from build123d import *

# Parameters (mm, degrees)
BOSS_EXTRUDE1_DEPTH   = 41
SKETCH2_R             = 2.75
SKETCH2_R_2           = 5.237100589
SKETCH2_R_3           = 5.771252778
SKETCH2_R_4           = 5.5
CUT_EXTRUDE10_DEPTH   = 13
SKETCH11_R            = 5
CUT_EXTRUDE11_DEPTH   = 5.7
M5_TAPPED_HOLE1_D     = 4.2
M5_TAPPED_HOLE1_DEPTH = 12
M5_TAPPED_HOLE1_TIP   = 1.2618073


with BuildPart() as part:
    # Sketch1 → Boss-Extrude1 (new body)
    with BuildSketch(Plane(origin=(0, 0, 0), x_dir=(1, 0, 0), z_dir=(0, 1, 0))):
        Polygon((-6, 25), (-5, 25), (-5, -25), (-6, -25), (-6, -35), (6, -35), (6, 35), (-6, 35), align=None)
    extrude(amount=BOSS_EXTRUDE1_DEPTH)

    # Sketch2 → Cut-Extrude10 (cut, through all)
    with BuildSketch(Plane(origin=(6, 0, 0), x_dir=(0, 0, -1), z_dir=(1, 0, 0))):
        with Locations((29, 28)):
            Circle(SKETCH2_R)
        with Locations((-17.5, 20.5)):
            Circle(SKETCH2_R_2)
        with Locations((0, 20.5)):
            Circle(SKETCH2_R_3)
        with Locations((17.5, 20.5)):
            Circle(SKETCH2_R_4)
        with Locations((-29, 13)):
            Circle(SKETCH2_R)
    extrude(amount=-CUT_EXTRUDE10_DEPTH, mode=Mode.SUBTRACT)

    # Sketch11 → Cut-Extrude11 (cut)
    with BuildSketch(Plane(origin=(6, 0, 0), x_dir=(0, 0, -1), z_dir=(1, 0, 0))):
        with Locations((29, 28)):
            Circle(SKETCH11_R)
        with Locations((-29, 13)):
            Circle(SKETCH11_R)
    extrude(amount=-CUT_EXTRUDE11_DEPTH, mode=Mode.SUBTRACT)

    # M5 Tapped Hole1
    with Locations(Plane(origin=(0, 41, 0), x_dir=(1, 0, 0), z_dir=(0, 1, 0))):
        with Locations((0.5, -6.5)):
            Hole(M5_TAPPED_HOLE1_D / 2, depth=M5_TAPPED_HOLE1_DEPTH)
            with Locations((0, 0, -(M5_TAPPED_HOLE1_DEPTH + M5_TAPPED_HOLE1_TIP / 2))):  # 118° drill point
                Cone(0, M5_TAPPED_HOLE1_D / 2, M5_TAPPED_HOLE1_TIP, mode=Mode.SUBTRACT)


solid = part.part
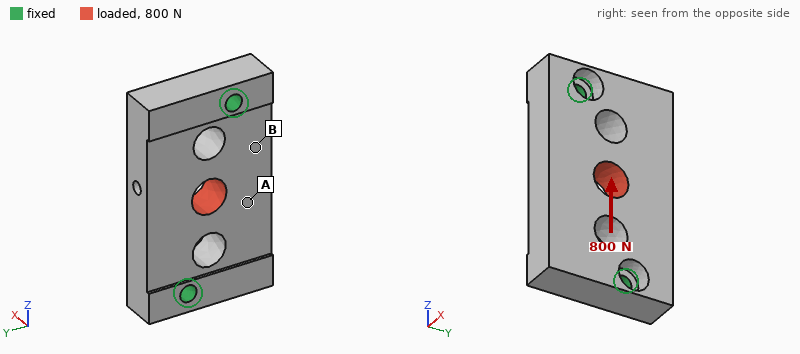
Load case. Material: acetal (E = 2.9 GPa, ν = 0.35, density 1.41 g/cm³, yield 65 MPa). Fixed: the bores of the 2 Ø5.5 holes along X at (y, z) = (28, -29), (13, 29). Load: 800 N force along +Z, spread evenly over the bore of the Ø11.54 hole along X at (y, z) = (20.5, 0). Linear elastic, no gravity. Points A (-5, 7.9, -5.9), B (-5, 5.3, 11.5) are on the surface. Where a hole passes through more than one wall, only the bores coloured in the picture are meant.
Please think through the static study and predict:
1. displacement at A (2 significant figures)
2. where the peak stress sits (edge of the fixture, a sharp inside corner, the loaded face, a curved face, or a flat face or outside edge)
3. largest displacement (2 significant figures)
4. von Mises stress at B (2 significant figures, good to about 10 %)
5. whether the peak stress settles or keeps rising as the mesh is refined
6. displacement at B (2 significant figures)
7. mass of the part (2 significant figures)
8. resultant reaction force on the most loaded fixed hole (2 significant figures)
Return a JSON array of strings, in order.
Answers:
["31 µm", "edge of the fixture", "42 µm", "2.0 MPa", "keeps rising", "25 µm", "39 g", "410 N"]
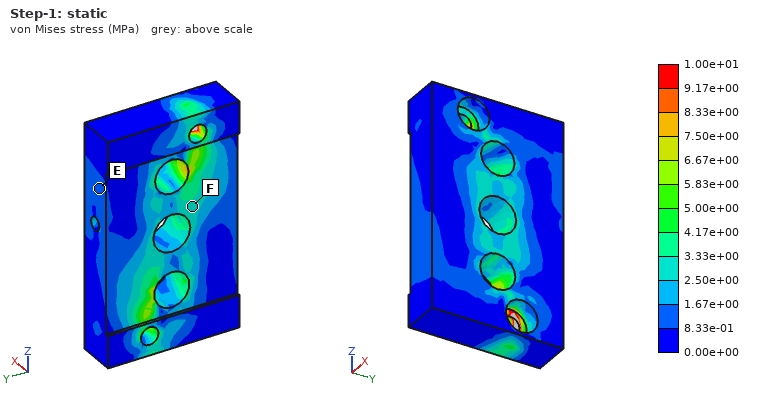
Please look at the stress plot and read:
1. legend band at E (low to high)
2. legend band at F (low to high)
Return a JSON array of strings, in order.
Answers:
["8.33e-01 to 1.67e+00 MPa", "2.50e+00 to 3.33e+00 MPa"]
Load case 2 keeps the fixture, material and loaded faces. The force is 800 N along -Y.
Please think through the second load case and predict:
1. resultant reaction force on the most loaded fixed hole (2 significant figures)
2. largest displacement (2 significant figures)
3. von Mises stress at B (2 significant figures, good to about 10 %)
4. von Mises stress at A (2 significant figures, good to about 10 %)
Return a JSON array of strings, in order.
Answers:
["400 N", "0.11 mm", "2.5 MPa", "2.1 MPa"]
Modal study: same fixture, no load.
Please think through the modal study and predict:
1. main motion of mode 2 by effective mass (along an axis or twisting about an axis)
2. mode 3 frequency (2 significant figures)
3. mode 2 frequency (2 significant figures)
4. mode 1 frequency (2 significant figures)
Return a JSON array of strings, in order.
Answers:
["along X", "3400 Hz", "2100 Hz", "1500 Hz"]
